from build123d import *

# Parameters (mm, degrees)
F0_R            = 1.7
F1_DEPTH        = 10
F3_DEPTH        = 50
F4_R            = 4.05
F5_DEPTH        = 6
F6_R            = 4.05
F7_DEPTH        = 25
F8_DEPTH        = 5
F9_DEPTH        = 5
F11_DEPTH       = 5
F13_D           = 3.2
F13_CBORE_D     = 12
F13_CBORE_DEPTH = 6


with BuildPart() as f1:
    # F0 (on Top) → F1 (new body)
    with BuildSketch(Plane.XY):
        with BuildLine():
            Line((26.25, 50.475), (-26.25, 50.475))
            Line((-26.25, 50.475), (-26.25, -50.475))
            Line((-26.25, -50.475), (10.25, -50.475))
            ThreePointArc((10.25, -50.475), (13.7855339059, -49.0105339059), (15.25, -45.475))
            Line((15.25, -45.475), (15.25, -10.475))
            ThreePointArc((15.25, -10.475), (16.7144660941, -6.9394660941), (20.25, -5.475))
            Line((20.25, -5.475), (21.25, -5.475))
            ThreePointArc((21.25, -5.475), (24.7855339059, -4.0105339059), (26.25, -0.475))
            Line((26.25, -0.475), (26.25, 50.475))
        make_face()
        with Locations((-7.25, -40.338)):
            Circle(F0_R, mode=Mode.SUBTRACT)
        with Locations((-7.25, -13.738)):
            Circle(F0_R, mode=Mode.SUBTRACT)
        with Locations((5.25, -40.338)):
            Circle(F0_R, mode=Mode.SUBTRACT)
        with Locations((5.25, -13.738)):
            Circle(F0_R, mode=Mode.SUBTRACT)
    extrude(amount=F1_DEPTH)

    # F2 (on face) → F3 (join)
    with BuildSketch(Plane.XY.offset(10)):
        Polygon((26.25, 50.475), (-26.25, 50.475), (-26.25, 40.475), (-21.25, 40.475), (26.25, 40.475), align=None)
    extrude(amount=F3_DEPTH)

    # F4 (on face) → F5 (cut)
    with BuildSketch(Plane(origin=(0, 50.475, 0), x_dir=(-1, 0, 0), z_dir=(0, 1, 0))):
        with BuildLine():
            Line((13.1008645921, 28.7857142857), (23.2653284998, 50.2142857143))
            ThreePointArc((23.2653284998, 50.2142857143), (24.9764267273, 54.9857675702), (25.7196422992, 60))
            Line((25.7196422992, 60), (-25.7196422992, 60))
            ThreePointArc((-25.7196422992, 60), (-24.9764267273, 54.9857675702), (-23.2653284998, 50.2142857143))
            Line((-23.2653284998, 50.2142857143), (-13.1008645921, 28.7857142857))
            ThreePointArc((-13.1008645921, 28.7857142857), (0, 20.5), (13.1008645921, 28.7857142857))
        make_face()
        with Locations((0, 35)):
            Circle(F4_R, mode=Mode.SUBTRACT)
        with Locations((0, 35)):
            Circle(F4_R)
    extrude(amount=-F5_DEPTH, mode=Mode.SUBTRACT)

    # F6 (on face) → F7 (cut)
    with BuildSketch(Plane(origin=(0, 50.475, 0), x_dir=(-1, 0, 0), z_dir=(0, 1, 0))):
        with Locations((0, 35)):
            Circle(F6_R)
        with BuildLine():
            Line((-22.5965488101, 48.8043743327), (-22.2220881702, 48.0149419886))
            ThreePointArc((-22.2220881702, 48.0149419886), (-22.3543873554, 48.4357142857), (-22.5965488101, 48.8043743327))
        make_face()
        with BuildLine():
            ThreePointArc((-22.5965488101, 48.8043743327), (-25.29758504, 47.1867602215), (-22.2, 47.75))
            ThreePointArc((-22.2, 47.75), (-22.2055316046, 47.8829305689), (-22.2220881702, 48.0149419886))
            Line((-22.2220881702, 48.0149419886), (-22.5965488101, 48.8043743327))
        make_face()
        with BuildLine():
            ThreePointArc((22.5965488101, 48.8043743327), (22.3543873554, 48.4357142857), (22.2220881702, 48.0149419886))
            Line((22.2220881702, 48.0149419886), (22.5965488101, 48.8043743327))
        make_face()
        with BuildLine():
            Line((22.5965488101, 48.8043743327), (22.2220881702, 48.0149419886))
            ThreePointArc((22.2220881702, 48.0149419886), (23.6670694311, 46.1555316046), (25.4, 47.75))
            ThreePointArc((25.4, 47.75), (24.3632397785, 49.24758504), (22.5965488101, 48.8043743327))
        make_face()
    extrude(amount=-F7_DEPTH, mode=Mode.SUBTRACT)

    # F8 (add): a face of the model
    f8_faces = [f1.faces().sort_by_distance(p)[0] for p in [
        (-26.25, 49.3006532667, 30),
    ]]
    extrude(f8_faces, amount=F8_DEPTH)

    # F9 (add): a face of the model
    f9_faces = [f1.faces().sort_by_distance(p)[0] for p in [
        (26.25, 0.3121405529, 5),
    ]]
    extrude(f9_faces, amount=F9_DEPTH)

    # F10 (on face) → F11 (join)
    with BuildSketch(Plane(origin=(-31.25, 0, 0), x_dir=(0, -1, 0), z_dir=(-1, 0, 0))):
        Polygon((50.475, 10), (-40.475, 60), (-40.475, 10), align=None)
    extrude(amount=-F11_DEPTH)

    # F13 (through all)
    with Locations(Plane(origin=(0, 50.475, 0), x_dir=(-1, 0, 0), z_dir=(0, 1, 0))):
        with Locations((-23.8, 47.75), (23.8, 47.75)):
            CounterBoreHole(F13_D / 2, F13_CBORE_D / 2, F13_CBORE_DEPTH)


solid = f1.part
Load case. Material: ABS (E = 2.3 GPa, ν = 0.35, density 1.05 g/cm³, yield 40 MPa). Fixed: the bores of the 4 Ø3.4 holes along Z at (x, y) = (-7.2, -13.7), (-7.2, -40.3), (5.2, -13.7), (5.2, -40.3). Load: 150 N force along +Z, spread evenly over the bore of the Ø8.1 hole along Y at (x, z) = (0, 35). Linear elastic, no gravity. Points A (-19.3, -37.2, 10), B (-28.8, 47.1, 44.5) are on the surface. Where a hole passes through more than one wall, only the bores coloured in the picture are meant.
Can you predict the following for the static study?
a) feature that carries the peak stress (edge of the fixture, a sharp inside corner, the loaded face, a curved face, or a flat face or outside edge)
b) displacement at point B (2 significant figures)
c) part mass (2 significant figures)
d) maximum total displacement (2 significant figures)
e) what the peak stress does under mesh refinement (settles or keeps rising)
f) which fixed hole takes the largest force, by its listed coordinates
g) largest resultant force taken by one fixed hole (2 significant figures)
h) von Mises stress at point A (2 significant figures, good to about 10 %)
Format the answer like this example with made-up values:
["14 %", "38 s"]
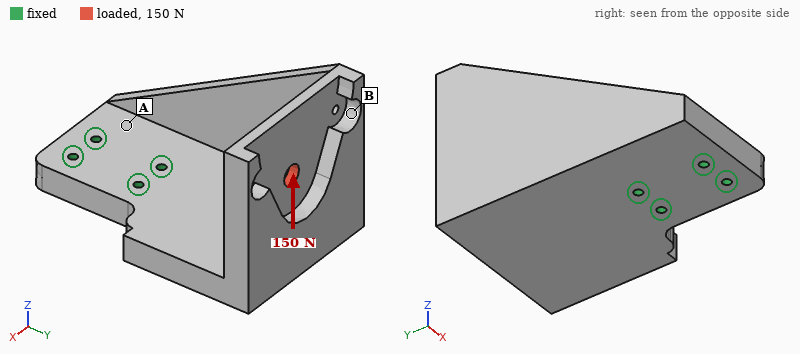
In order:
["edge of the fixture", "0.60 mm", "93 g", "0.95 mm", "keeps rising", "(-7.2, -13.7)", "240 N", "2.5 MPa"]
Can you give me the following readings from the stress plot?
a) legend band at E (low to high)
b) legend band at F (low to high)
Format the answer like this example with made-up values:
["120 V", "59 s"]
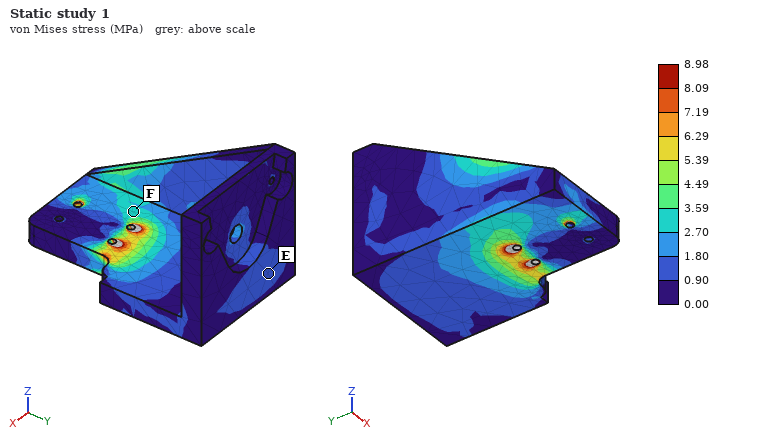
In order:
["0.90 to 1.80 MPa", "2.70 to 3.59 MPa"]
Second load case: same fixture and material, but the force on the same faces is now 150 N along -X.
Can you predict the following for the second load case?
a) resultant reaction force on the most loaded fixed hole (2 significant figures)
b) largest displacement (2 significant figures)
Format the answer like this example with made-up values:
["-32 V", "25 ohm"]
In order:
["320 N", "0.94 mm"]
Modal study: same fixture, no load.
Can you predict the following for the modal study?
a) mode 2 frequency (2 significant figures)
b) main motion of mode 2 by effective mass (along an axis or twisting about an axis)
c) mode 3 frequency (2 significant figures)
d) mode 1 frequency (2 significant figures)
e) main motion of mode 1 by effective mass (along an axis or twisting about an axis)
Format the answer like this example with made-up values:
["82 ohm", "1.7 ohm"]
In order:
["420 Hz", "along X", "890 Hz", "360 Hz", "along Z"]
